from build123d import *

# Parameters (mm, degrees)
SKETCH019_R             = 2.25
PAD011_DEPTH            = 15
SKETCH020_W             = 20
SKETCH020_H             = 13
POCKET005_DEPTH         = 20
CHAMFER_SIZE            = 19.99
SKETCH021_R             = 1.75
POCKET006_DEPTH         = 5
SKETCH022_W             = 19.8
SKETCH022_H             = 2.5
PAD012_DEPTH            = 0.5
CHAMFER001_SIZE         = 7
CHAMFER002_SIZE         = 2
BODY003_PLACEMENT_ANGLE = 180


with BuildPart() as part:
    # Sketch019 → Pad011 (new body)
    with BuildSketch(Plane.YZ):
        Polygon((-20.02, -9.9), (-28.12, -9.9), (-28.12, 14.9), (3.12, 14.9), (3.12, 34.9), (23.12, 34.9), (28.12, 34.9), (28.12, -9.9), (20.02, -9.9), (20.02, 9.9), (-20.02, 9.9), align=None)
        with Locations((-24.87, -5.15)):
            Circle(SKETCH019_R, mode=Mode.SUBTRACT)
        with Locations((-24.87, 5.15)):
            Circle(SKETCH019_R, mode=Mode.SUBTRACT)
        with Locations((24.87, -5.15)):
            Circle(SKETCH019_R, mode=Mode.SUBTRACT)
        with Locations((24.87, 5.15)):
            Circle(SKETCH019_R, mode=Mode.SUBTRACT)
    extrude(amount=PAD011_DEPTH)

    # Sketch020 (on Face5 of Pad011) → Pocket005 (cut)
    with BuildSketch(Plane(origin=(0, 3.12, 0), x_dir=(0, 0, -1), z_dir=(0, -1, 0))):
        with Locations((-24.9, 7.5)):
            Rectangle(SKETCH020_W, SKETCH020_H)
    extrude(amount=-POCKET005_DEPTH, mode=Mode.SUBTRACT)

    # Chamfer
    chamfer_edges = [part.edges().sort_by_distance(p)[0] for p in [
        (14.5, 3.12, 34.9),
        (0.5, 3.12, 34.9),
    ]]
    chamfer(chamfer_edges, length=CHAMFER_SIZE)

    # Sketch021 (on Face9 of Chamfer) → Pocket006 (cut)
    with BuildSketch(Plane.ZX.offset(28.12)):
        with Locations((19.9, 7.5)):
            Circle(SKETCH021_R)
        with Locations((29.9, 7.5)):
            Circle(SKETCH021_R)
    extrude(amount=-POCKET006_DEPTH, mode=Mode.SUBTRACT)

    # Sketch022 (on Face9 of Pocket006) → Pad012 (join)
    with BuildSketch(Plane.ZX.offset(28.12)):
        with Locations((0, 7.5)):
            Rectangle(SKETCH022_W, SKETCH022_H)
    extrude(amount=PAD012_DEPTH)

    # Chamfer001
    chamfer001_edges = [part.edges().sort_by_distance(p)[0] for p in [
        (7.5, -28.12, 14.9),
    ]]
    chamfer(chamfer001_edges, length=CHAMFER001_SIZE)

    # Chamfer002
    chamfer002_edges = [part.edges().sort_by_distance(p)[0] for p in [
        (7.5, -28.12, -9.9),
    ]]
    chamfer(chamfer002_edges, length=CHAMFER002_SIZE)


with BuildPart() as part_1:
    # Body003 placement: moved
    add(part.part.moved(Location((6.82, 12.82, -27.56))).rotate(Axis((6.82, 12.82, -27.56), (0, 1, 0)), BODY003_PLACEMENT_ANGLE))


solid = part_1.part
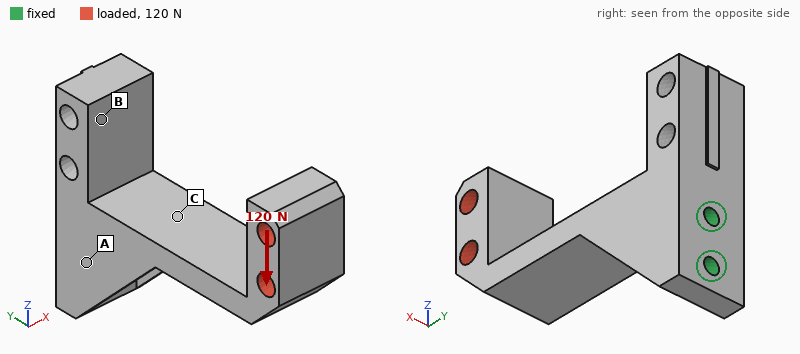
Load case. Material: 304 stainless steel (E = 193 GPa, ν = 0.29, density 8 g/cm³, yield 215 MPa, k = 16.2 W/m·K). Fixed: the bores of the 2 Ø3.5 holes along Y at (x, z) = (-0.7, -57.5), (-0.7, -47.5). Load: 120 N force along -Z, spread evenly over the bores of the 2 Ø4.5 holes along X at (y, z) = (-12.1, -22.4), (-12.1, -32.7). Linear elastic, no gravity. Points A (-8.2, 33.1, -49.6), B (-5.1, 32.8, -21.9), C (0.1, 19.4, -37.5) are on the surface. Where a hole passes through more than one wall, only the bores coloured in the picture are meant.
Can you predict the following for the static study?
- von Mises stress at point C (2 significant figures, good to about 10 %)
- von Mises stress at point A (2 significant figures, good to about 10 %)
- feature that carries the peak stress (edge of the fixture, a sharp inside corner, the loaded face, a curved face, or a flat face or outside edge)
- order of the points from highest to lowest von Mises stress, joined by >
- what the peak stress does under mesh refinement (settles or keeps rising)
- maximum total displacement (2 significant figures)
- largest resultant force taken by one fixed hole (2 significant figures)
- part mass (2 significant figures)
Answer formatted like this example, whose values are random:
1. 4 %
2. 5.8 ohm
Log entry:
1. 47 MPa
2. 16 MPa
3. a sharp inside corner
4. C > A > B
5. keeps rising
6. 0.11 mm
7. 390 N
8. 76 g
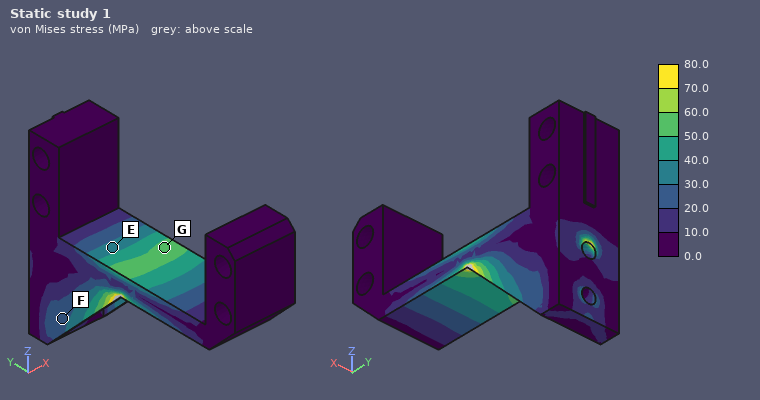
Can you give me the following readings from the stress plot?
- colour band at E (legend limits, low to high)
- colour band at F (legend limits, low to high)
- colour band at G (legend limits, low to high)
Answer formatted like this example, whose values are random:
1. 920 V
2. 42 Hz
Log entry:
1. 30.0 to 40.0 MPa
2. 20.0 to 30.0 MPa
3. 50.0 to 60.0 MPa
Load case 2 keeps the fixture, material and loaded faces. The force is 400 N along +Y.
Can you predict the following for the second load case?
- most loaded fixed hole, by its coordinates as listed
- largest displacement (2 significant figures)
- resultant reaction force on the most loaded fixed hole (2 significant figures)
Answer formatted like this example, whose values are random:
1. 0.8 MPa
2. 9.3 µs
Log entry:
1. (-0.7, -47.5)
2. 0.20 mm
3. 820 N
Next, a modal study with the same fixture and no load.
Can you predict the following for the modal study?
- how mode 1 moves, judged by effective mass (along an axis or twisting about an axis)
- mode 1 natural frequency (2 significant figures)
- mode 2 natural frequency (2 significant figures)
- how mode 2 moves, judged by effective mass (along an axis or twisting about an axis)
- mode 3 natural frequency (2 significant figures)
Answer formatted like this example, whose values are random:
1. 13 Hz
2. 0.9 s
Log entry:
1. along Z
2. 1300 Hz
3. 1800 Hz
4. along X
5. 3800 Hz
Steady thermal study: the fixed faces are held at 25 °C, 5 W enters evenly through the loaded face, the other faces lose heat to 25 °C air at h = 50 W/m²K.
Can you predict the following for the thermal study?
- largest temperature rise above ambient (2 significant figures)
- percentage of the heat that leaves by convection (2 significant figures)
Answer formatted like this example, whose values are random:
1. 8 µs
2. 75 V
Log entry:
1. 62 K
2. 92 %
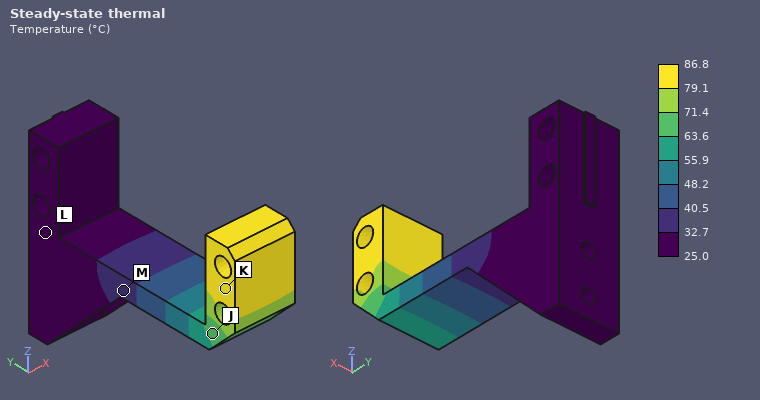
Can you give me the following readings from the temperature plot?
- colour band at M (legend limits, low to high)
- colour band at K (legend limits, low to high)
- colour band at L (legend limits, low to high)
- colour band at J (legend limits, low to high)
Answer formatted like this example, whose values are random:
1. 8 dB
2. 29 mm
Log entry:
1. 32.7 to 40.5 °C
2. 79.1 to 86.8 °C
3. 25.0 to 32.7 °C
4. 63.6 to 71.4 °C
